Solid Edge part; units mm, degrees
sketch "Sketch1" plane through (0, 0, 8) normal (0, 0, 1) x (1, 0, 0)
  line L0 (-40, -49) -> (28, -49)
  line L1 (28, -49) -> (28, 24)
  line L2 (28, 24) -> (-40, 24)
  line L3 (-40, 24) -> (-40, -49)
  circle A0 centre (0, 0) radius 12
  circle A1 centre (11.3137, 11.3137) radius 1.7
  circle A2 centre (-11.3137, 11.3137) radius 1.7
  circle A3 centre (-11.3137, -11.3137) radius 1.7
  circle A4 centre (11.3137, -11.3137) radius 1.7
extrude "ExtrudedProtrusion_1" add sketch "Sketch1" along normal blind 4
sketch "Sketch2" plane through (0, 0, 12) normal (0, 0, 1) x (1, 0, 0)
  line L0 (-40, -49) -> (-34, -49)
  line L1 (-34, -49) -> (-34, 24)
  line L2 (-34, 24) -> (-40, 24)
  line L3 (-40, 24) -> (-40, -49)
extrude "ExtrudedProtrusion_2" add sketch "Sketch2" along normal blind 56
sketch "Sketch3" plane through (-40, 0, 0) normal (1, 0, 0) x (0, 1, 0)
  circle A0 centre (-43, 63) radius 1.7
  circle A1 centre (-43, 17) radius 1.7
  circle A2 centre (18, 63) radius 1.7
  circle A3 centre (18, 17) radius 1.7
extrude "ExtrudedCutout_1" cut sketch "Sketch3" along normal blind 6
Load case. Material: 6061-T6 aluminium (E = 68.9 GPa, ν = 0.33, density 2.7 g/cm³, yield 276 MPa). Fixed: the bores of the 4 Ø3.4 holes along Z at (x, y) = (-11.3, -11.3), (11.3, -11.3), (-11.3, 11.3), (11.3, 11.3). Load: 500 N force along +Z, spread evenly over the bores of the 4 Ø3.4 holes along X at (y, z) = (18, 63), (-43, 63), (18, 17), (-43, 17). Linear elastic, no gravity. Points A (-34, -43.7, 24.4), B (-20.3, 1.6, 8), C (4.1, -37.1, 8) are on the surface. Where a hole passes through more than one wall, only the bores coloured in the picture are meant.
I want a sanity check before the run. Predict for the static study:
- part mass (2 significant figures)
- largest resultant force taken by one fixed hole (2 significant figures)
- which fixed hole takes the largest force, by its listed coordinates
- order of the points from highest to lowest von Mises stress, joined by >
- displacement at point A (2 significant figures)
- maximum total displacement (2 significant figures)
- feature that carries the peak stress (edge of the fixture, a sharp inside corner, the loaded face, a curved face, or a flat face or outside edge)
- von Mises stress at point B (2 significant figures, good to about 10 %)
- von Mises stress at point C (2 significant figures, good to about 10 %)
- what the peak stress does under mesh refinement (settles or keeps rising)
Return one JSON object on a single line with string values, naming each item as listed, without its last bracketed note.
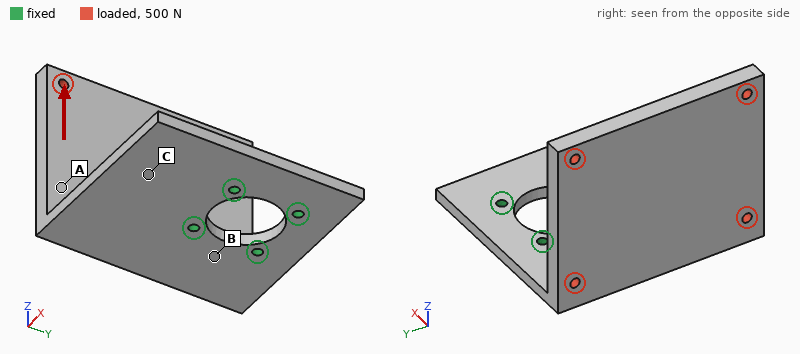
{"part mass": "110 g", "largest resultant force taken by one fixed hole": "580 N", "which fixed hole takes the largest force, by its listed coordinates": "(-11.3, -11.3)", "order of the points from highest to lowest von Mises stress, joined by >": "B > C > A", "displacement at point A": "0.22 mm", "maximum total displacement": "0.52 mm", "feature that carries the peak stress": "edge of the fixture", "von Mises stress at point B": "41 MPa", "von Mises stress at point C": "17 MPa", "what the peak stress does under mesh refinement": "keeps rising"}
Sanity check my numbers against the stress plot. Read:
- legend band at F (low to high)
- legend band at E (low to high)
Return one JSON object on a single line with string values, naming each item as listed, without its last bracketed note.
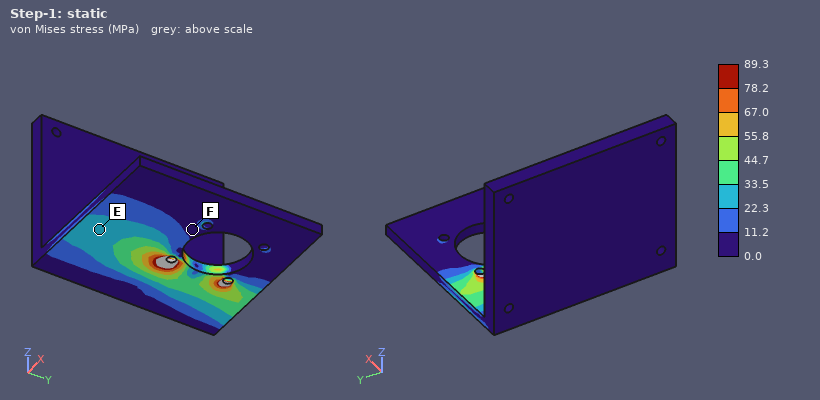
{"legend band at F": "0.0 to 11.2 MPa", "legend band at E": "22.3 to 33.5 MPa"}
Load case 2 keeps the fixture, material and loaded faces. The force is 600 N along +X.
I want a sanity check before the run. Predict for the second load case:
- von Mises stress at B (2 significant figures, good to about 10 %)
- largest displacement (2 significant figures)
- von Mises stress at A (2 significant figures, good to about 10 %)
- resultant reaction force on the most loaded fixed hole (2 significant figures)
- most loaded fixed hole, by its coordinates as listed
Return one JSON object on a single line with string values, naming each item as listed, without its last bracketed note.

{"von Mises stress at B": "79 MPa", "largest displacement": "1.3 mm", "von Mises stress at A": "21 MPa", "resultant reaction force on the most loaded fixed hole": "450 N", "most loaded fixed hole, by its coordinates as listed": "(-11.3, -11.3)"}
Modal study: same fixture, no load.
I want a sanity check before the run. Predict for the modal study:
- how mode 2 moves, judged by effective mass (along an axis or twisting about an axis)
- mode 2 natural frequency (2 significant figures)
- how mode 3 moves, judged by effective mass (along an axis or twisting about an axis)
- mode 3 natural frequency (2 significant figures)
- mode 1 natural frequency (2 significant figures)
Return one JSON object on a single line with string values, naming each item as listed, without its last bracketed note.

{"how mode 2 moves, judged by effective mass": "along Y", "mode 2 natural frequency": "860 Hz", "how mode 3 moves, judged by effective mass": "along Z", "mode 3 natural frequency": "2000 Hz", "mode 1 natural frequency": "490 Hz"}
